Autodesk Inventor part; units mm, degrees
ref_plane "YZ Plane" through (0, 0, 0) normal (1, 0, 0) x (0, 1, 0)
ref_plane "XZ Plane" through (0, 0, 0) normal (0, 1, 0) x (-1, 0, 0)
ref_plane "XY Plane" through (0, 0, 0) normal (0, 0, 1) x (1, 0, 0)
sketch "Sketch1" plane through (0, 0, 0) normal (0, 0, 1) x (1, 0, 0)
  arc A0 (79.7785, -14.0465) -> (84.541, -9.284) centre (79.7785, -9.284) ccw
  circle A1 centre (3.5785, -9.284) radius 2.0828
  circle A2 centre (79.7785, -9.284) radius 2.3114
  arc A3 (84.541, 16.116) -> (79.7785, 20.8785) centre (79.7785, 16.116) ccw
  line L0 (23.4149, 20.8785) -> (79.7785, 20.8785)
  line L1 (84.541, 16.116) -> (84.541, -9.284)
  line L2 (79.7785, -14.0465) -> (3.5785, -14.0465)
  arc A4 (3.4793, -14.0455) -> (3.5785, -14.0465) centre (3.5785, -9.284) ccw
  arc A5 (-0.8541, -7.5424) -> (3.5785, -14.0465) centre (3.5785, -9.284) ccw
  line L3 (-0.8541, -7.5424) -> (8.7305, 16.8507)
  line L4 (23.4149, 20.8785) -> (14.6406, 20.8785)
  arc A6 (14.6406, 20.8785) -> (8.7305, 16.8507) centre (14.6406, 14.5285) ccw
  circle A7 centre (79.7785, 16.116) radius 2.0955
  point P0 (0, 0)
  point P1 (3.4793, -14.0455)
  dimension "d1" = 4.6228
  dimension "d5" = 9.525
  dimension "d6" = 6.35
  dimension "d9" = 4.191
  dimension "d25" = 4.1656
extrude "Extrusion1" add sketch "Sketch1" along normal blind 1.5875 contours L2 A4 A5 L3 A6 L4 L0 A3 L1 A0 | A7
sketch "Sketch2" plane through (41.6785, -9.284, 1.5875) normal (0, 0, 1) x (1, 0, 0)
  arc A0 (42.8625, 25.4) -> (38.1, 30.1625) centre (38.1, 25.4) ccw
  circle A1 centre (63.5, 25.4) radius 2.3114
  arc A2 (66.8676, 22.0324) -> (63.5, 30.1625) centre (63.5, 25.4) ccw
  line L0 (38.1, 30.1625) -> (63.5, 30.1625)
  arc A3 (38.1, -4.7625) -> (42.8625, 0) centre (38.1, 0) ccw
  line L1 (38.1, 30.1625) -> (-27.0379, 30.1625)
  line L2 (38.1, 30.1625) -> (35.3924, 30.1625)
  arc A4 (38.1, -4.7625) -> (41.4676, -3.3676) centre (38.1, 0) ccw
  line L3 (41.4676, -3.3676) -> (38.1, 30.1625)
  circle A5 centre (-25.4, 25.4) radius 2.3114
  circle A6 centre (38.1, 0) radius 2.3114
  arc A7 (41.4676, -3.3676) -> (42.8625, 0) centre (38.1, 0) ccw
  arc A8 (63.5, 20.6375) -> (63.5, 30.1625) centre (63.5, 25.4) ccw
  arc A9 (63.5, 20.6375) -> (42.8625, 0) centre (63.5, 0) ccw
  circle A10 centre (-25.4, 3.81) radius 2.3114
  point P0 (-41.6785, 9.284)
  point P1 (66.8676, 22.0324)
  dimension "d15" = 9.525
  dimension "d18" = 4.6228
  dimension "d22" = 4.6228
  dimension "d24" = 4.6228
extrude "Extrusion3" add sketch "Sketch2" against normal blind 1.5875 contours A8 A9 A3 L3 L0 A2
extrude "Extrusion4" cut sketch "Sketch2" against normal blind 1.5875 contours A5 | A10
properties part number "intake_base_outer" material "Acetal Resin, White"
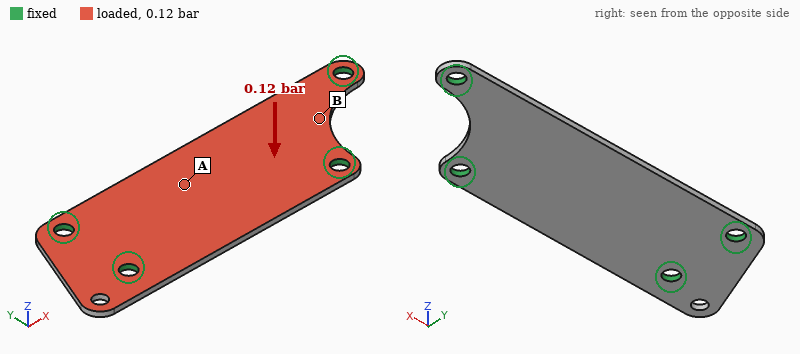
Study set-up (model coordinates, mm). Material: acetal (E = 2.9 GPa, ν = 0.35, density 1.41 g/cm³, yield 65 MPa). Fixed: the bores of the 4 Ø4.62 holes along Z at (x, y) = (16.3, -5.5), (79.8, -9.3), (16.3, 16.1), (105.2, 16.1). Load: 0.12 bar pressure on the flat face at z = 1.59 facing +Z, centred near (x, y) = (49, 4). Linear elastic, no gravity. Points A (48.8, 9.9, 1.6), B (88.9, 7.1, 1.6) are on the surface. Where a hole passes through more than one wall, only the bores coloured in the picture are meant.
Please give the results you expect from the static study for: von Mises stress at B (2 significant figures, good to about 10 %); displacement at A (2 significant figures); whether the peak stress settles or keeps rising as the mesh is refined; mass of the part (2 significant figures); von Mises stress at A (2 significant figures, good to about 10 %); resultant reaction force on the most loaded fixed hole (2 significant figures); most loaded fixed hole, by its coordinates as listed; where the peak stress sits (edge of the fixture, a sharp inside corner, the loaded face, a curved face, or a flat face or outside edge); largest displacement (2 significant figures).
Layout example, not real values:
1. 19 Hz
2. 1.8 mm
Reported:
1. 2.3 MPa
2. 0.78 mm
3. keeps rising
4. 6.8 g
5. 5.2 MPa
6. 13 N
7. (79.8, -9.3)
8. edge of the fixture
9. 1.1 mm
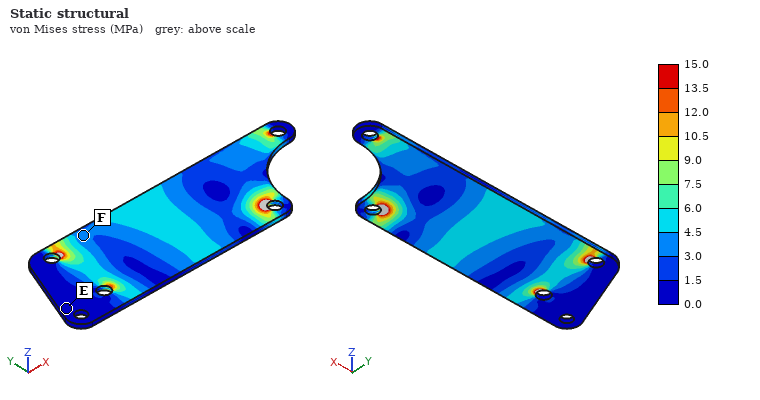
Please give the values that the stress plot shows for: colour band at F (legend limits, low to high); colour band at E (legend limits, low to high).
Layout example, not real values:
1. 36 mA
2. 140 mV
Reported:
1. 3.0 to 4.5 MPa
2. 0.0 to 1.5 MPa
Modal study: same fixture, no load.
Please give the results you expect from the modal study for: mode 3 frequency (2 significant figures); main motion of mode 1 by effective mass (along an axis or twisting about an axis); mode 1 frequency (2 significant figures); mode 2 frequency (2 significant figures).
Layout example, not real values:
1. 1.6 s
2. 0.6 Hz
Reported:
1. 1200 Hz
2. along Z
3. 470 Hz
4. 770 Hz
